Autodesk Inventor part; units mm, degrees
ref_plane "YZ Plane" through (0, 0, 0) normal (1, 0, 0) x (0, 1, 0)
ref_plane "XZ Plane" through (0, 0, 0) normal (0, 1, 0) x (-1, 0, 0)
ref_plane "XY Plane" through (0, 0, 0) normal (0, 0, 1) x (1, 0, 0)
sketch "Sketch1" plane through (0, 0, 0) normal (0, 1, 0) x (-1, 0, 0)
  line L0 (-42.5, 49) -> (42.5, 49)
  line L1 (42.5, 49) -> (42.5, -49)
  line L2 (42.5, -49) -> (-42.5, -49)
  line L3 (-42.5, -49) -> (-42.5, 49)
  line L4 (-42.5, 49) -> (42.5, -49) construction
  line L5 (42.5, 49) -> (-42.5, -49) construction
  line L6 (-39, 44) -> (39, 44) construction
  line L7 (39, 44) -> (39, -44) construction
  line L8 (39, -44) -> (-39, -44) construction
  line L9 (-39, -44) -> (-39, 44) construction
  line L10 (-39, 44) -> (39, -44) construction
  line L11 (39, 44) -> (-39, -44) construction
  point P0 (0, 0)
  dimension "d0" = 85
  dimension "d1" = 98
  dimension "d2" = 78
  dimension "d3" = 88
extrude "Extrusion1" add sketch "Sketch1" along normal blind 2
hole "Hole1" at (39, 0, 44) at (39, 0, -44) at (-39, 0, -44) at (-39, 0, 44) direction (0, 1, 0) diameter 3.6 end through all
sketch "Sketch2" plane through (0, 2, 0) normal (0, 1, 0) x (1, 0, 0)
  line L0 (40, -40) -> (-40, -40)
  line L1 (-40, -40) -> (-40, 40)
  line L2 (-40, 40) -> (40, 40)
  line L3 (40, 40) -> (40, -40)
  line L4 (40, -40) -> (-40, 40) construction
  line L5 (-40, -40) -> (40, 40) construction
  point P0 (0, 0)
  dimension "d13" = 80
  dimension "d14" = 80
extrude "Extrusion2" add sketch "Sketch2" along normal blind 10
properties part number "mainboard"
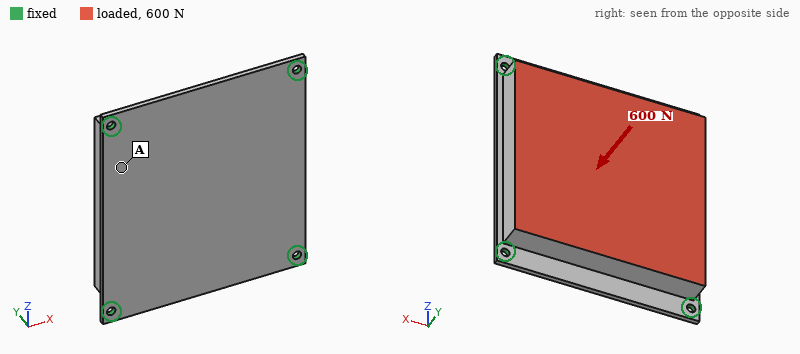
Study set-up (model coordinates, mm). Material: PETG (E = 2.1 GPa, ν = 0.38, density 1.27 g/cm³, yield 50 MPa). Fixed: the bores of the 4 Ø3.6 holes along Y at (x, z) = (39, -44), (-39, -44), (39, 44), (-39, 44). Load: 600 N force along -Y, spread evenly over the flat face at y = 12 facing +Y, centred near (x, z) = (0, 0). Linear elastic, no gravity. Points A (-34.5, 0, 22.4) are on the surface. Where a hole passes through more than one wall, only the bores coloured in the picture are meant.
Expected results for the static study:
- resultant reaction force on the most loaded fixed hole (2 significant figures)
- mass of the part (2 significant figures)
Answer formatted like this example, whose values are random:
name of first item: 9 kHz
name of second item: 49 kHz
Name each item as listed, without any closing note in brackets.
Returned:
resultant reaction force on the most loaded fixed hole: 240 N
mass of the part: 100 g
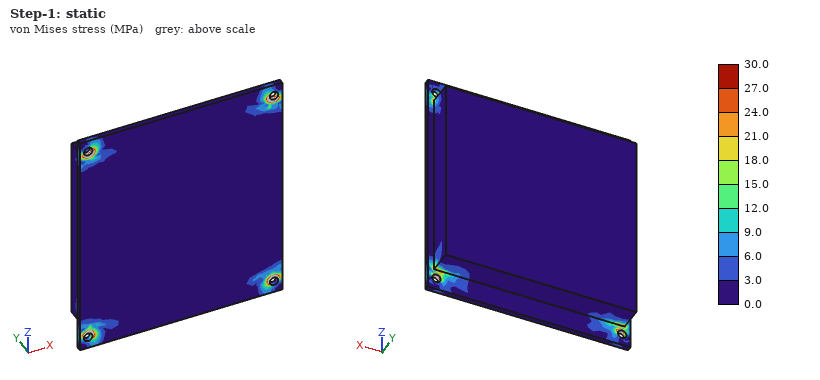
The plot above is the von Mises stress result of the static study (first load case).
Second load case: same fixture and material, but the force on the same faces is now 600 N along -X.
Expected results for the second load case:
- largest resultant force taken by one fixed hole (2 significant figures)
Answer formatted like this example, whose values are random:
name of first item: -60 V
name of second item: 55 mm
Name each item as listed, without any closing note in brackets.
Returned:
largest resultant force taken by one fixed hole: 170 N
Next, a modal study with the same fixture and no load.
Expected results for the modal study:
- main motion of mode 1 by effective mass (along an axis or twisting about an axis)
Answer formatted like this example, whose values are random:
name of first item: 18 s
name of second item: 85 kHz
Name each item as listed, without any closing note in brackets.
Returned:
main motion of mode 1 by effective mass: along Y
